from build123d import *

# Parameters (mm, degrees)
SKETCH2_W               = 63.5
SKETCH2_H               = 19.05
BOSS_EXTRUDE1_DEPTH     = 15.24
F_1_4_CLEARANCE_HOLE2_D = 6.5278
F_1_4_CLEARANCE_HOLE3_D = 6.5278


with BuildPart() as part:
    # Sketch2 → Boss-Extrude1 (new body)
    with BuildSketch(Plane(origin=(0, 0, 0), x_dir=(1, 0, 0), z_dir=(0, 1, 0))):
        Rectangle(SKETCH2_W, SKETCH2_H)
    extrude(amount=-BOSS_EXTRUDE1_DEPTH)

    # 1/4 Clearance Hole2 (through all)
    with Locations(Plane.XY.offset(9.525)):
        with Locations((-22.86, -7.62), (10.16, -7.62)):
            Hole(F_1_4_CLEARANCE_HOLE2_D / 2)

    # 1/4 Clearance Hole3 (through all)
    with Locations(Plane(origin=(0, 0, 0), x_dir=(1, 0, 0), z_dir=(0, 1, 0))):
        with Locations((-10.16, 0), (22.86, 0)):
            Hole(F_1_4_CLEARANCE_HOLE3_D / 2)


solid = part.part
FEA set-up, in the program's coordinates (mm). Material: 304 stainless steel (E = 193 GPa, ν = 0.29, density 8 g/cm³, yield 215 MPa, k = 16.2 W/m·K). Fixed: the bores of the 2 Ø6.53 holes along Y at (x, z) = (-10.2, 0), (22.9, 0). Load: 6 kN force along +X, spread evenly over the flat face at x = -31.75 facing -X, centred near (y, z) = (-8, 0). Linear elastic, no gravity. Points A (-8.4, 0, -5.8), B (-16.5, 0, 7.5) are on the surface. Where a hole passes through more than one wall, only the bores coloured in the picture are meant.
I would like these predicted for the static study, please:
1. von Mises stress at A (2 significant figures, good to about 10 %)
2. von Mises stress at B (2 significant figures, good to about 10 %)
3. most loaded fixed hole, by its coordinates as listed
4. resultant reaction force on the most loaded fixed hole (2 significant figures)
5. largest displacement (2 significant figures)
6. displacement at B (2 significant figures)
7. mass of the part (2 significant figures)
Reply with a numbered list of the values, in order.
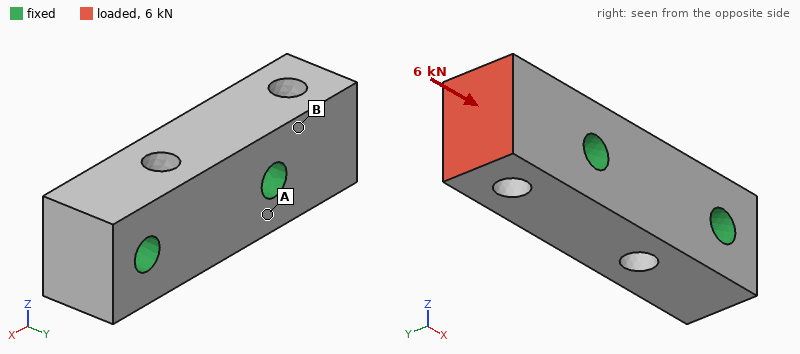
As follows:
1. 10 MPa
2. 26 MPa
3. (-10.2, 0)
4. 5.7 kN
5. 3.7 µm
6. 1.2 µm
7. 130 g
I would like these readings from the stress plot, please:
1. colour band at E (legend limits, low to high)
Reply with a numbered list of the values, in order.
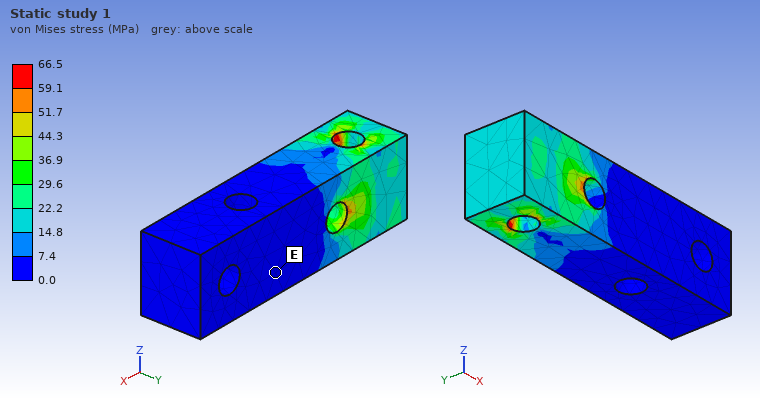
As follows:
1. 0.0 to 7.4 MPa
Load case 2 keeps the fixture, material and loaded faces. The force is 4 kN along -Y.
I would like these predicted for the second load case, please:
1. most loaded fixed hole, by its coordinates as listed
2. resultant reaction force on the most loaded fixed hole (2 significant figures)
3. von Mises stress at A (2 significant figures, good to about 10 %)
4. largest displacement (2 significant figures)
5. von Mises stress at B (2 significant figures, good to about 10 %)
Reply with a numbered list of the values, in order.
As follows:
1. (-10.2, 0)
2. 4.2 kN
3. 36 MPa
4. 22 µm
5. 83 MPa
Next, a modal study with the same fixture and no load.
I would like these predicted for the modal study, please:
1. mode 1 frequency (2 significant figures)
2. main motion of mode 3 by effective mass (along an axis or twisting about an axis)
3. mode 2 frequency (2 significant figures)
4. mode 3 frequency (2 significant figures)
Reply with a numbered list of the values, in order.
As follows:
1. 19 kHz
2. twisting about X
3. 19 kHz
4. 31 kHz
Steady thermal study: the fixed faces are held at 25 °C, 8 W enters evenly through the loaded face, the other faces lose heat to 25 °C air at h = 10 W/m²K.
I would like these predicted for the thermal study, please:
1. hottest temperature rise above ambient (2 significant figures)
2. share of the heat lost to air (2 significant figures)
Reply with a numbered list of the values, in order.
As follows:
1. 43 K
2. 4.8 %
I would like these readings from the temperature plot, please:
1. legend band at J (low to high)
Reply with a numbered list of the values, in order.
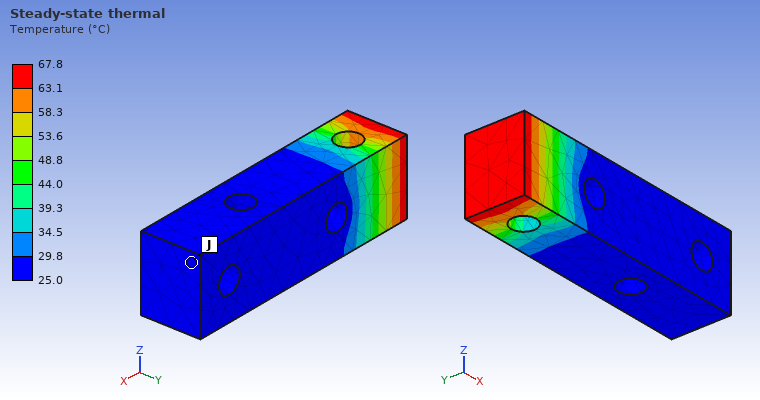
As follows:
1. 25.0 to 29.8 °C
